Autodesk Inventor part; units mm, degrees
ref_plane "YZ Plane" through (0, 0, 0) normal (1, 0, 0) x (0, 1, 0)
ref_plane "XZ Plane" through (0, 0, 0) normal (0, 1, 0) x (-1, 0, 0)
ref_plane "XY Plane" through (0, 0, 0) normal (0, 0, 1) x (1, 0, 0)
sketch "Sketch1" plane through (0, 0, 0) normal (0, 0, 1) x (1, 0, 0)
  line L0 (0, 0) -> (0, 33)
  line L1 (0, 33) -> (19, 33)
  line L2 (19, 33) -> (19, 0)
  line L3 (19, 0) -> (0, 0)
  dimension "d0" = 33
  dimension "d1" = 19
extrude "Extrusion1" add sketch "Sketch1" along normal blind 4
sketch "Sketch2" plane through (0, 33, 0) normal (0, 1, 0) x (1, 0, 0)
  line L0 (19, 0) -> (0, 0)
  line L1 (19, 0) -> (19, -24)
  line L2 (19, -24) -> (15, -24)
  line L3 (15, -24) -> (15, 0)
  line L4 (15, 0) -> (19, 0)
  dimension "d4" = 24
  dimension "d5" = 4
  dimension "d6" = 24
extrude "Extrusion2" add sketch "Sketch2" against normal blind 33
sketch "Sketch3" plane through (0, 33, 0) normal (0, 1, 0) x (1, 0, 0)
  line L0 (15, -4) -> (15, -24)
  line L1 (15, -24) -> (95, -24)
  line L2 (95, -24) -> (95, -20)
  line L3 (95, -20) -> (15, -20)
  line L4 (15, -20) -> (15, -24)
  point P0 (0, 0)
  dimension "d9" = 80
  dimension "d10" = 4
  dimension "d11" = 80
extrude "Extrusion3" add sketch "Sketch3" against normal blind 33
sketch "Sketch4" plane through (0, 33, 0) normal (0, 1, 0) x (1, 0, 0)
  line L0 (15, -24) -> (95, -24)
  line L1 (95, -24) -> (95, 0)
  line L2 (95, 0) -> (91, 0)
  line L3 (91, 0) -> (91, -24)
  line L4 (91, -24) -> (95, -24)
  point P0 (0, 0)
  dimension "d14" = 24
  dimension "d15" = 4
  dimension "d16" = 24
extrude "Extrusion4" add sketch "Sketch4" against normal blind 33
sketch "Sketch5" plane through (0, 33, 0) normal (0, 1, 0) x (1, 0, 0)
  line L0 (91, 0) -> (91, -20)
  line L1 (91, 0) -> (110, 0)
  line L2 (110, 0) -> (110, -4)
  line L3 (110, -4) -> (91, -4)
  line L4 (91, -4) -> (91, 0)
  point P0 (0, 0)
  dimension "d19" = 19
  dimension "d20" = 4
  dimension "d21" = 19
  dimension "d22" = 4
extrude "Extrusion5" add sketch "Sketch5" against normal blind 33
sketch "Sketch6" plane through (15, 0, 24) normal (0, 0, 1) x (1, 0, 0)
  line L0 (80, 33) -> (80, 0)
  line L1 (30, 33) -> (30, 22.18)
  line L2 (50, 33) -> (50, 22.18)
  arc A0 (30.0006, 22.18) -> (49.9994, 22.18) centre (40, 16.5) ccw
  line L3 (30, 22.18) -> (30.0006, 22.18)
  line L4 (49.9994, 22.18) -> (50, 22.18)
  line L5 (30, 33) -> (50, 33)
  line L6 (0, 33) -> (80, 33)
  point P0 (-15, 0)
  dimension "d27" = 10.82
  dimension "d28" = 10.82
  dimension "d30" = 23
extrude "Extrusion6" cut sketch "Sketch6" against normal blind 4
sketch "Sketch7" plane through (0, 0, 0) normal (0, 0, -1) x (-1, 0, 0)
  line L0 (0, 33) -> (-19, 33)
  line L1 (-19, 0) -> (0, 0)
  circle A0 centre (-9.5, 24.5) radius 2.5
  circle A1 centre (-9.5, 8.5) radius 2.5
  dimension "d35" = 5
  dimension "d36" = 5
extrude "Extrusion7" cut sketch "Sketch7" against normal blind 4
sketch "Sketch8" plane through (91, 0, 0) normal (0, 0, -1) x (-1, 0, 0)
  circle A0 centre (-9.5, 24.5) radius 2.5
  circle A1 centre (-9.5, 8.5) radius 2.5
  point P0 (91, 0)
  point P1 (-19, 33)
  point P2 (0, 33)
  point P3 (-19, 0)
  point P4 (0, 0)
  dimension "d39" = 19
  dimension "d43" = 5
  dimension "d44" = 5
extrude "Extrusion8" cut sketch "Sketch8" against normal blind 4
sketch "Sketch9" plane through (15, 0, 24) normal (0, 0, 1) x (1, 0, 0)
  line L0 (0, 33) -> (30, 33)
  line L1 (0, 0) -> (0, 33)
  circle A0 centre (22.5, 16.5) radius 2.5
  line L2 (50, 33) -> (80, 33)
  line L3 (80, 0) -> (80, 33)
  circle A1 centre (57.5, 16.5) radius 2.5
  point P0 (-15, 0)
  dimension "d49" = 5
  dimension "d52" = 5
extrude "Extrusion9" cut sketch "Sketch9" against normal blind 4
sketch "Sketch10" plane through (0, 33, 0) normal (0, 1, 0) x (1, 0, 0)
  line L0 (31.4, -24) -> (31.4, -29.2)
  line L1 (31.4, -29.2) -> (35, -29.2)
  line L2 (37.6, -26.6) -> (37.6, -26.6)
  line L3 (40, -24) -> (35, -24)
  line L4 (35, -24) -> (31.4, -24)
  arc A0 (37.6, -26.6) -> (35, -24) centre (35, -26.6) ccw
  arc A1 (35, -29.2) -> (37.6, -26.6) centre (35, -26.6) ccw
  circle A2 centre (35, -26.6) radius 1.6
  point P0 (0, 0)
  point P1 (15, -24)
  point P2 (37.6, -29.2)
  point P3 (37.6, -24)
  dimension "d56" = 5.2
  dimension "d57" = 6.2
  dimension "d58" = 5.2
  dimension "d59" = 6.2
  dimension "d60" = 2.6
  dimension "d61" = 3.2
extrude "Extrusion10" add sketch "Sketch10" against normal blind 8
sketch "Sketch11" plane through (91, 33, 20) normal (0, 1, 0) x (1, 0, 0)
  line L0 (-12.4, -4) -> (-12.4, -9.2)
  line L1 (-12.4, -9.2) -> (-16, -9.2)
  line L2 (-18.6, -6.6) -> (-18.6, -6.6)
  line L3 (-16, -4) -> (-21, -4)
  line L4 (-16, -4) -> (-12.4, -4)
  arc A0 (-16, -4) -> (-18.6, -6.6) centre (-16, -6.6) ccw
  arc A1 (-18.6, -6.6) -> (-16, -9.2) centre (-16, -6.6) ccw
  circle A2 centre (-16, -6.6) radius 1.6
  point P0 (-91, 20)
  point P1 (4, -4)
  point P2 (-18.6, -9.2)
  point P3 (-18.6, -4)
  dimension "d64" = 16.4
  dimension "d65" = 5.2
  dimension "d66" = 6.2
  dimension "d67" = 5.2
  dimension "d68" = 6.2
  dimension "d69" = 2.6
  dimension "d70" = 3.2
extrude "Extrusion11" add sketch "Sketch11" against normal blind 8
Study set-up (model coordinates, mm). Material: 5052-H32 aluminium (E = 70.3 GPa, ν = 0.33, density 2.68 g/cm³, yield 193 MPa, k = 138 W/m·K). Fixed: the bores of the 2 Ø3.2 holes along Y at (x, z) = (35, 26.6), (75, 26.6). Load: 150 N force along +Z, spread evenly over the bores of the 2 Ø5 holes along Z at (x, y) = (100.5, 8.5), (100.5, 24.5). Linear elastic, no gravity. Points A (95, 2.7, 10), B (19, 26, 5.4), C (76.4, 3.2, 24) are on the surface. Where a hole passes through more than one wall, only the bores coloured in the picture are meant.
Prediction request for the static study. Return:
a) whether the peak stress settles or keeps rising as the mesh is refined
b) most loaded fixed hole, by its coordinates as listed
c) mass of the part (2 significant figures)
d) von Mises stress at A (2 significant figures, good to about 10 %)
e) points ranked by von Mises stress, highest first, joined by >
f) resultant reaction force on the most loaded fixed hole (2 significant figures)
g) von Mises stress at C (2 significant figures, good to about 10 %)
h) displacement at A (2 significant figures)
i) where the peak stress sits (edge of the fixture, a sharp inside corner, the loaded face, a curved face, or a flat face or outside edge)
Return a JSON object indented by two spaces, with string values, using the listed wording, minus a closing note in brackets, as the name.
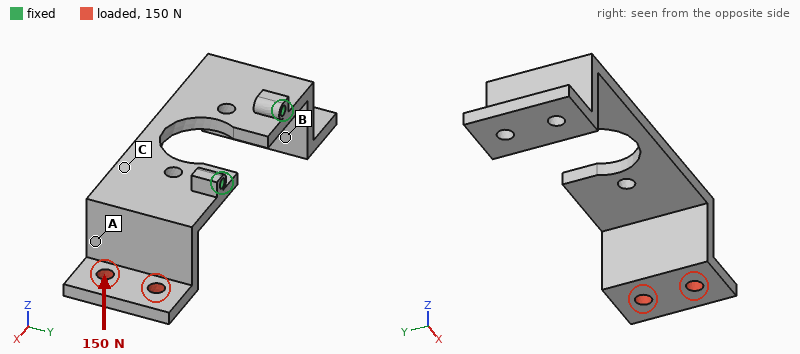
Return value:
{
  "whether the peak stress settles or keeps rising as the mesh is refined": "keeps rising",
  "most loaded fixed hole, by its coordinates as listed": "(75, 26.6)",
  "mass of the part": "47 g",
  "von Mises stress at A": "13 MPa",
  "points ranked by von Mises stress, highest first, joined by >": "C > A > B",
  "resultant reaction force on the most loaded fixed hole": "180 N",
  "von Mises stress at C": "22 MPa",
  "displacement at A": "0.20 mm",
  "where the peak stress sits": "a sharp inside corner"
}
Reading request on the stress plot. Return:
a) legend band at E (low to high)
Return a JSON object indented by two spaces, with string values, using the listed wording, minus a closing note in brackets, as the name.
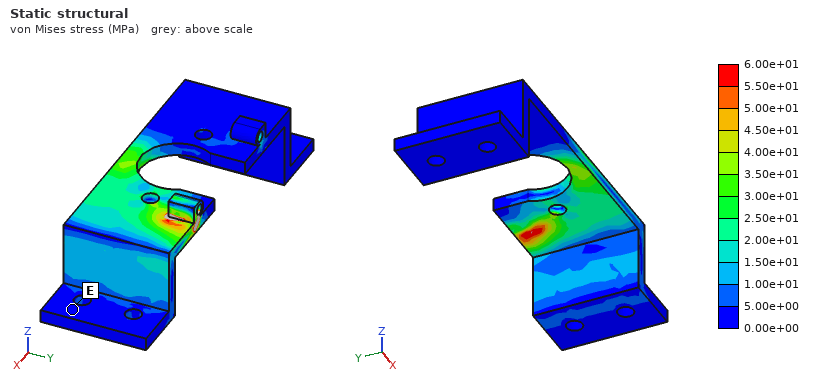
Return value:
{
  "legend band at E": "0.00e+00 to 5.00e+00 MPa"
}
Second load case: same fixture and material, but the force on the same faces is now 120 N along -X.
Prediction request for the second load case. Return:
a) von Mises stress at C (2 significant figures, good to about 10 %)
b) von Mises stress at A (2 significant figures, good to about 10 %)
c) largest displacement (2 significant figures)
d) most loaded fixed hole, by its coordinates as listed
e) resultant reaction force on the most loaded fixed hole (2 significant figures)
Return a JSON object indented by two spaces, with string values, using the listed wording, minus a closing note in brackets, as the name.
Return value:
{
  "von Mises stress at C": "18 MPa",
  "von Mises stress at A": "11 MPa",
  "largest displacement": "0.26 mm",
  "most loaded fixed hole, by its coordinates as listed": "(75, 26.6)",
  "resultant reaction force on the most loaded fixed hole": "88 N"
}
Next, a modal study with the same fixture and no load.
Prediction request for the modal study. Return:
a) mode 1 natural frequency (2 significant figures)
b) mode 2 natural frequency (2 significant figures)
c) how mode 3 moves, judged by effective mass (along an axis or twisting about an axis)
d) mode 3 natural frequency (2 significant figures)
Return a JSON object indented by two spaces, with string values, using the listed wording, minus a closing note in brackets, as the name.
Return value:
{
  "mode 1 natural frequency": "1100 Hz",
  "mode 2 natural frequency": "1100 Hz",
  "how mode 3 moves, judged by effective mass": "along Y",
  "mode 3 natural frequency": "1700 Hz"
}
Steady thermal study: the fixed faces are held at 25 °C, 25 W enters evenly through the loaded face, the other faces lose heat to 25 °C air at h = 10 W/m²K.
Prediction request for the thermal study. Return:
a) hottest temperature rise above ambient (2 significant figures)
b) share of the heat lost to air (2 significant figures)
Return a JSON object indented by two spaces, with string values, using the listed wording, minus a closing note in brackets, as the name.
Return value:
{
  "hottest temperature rise above ambient": "79 K",
  "share of the heat lost to air": "10 %"
}
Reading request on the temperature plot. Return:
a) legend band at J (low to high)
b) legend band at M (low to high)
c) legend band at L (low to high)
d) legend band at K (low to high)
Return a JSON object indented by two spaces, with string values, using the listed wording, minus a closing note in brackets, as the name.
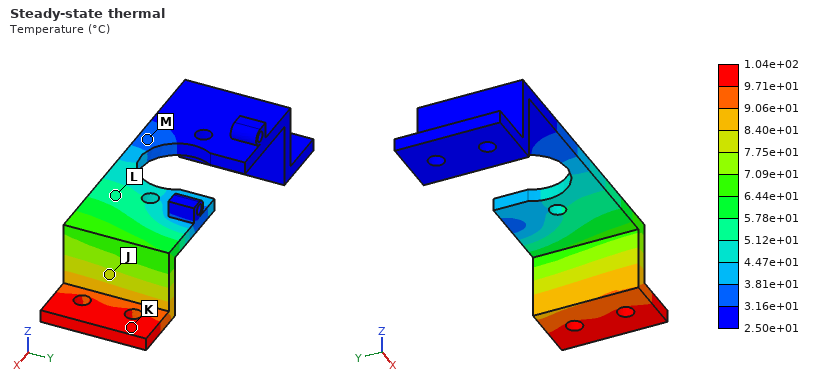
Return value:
{
  "legend band at J": "7.75e+01 to 8.40e+01 °C",
  "legend band at M": "3.16e+01 to 3.81e+01 °C",
  "legend band at L": "5.12e+01 to 5.78e+01 °C",
  "legend band at K": "9.71e+01 to 1.04e+02 °C"
}
